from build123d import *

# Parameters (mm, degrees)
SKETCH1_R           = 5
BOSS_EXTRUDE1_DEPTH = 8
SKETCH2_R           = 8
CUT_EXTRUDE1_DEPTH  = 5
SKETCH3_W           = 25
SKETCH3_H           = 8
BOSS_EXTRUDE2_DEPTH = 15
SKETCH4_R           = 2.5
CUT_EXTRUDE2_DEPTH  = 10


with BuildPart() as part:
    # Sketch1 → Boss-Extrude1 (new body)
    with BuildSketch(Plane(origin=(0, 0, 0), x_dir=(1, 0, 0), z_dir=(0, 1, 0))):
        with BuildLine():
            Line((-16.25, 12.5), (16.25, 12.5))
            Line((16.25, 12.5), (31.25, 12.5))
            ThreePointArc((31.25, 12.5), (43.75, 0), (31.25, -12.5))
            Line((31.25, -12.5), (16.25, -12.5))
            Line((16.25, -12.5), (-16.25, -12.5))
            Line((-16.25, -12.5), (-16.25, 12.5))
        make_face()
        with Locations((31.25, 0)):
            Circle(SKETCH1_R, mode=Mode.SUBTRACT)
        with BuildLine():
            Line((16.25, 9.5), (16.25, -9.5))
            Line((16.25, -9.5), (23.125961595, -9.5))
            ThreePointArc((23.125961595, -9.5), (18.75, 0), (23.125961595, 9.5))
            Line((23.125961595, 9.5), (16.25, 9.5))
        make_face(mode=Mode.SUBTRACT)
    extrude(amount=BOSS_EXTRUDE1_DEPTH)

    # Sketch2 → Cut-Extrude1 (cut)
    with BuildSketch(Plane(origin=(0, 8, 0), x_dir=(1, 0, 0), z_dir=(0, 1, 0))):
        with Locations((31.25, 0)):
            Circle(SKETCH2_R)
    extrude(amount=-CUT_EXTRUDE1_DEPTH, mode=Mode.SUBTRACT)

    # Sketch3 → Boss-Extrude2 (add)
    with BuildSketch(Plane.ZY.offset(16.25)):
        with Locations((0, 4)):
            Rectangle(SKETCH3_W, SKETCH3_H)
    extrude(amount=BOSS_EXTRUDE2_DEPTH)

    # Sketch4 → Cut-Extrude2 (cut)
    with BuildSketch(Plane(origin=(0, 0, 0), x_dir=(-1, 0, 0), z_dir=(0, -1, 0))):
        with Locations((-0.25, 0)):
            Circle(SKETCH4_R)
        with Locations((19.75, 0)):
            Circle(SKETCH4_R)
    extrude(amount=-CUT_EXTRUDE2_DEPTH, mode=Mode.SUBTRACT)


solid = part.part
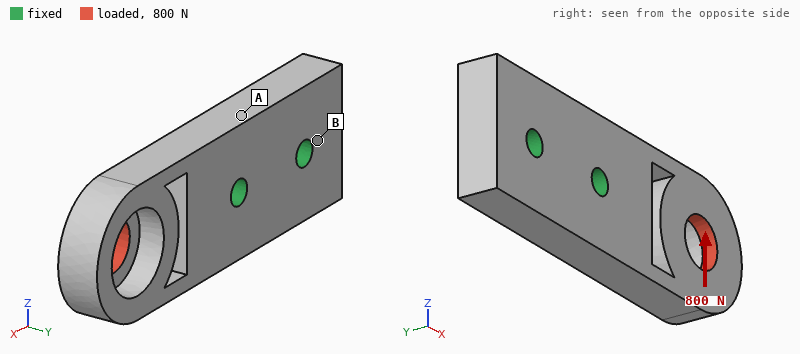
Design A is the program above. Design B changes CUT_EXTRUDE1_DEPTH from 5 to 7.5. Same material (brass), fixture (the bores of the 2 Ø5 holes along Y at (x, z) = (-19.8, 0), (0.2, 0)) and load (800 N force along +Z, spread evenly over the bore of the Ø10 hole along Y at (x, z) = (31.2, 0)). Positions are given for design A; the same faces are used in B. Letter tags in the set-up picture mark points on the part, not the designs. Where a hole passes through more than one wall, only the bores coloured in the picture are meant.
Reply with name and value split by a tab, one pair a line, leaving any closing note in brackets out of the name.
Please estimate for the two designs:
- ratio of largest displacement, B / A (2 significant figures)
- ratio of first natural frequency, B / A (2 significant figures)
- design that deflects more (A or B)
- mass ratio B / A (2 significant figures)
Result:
ratio of largest displacement, B / A	1.2
ratio of first natural frequency, B / A	1.1
design that deflects more	B
mass ratio B / A	0.98
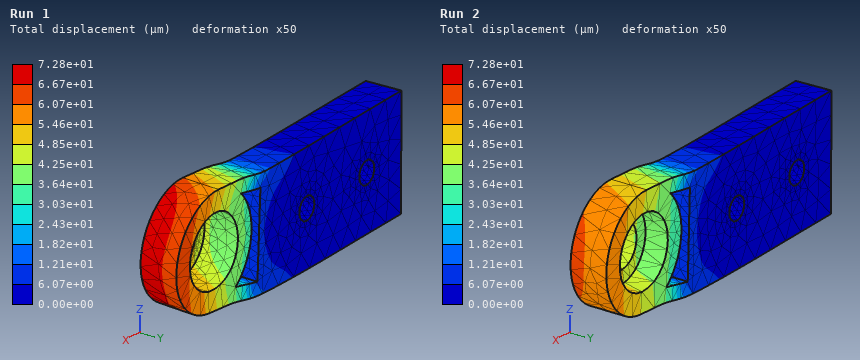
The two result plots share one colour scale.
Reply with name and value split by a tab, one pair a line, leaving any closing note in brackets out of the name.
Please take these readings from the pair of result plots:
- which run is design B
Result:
which run is design B	Run 1
